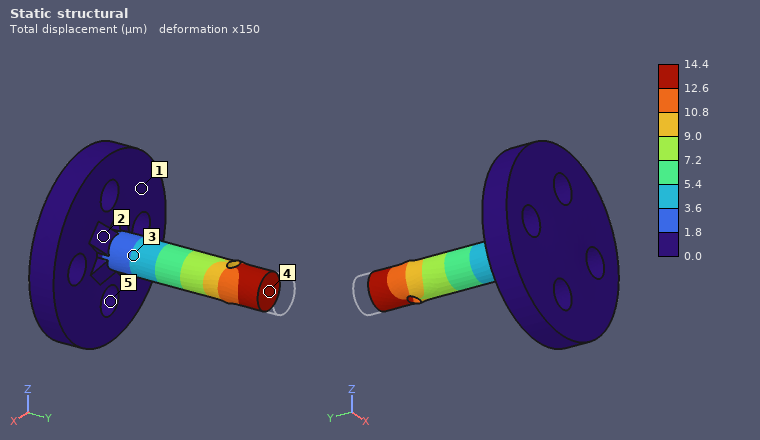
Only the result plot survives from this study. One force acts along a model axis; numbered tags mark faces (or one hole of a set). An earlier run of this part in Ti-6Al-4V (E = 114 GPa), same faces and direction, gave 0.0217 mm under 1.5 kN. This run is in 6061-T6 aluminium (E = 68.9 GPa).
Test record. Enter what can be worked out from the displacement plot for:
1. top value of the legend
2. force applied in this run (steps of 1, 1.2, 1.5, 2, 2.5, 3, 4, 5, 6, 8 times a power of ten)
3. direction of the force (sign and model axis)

14.4 µm
600 N
-Y
